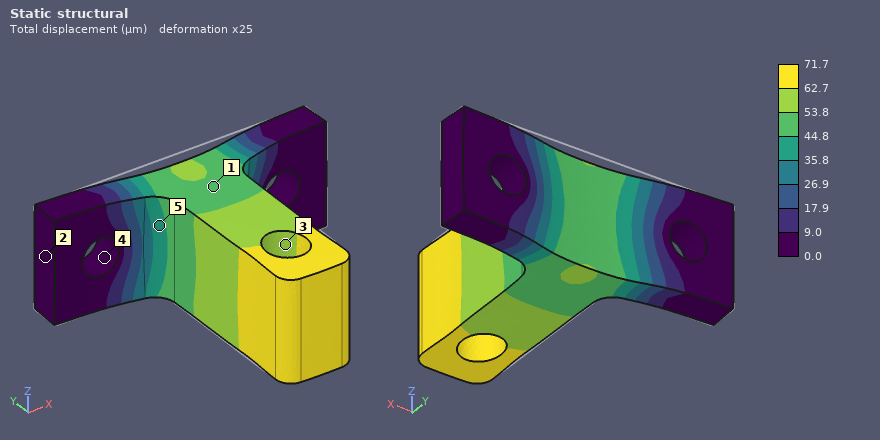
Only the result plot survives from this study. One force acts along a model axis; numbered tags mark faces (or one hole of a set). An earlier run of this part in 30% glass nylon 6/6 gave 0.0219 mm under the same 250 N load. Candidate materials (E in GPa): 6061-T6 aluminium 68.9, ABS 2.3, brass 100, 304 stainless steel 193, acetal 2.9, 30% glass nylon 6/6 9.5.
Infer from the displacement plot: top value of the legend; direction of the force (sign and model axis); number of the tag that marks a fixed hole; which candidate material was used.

71.7 µm
-Y
4
acetal
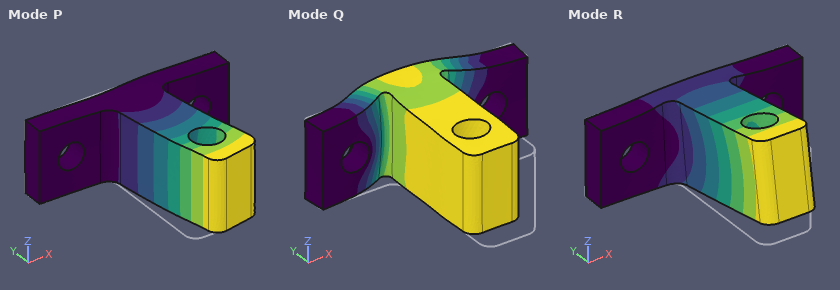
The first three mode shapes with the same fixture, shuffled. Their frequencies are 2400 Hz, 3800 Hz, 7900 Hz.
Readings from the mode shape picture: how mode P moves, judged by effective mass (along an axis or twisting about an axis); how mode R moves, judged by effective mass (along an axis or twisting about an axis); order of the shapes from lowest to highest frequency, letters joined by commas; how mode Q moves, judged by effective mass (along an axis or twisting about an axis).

along X
along Z
R, P, Q
along Y
